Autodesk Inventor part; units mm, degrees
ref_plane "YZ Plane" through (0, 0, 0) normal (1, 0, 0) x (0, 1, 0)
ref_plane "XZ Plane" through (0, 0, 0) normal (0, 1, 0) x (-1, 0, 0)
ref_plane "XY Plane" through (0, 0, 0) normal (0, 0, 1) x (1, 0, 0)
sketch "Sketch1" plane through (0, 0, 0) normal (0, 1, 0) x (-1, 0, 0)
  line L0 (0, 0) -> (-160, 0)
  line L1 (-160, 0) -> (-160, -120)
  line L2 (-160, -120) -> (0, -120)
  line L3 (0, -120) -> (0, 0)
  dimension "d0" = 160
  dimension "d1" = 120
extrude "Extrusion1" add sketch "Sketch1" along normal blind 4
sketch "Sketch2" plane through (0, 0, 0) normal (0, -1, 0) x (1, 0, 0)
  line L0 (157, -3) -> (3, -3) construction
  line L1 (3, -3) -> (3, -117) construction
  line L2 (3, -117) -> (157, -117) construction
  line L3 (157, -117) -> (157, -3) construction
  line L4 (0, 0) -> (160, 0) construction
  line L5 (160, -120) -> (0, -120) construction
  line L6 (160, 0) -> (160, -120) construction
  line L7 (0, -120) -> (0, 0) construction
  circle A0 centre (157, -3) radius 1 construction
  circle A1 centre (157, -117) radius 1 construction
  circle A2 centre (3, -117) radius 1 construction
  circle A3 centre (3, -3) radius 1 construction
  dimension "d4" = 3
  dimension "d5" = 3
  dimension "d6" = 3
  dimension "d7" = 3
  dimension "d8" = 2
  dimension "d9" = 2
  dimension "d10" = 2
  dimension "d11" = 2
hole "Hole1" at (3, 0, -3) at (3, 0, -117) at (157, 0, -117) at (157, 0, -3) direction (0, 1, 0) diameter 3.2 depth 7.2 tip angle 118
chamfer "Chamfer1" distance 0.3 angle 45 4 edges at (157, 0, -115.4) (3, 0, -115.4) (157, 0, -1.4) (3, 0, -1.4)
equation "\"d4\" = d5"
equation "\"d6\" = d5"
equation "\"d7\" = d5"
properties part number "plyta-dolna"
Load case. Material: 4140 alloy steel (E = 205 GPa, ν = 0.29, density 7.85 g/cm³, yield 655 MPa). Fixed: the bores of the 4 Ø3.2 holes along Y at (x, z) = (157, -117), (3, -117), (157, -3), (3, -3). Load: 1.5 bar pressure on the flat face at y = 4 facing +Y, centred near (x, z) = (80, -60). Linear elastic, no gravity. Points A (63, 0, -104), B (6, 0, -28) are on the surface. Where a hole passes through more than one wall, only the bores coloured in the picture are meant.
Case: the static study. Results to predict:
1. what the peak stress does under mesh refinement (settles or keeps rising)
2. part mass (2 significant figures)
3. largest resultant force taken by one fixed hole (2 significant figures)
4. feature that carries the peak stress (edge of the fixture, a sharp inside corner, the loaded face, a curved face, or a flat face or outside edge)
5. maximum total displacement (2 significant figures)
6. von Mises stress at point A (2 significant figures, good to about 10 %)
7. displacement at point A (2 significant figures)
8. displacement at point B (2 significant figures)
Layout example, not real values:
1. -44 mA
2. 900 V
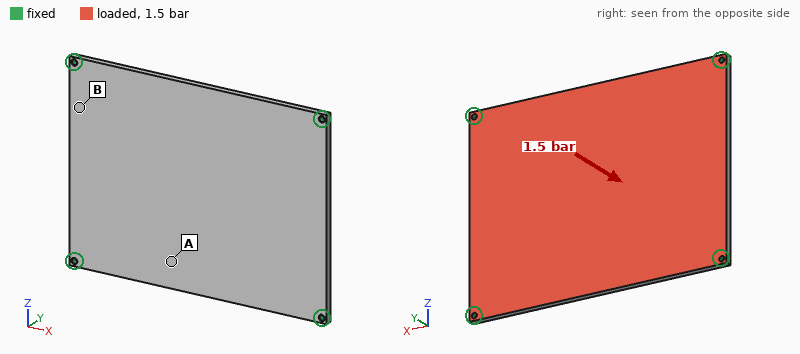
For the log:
1. keeps rising
2. 600 g
3. 720 N
4. edge of the fixture
5. 0.50 mm
6. 80 MPa
7. 0.42 mm
8. 0.095 mm
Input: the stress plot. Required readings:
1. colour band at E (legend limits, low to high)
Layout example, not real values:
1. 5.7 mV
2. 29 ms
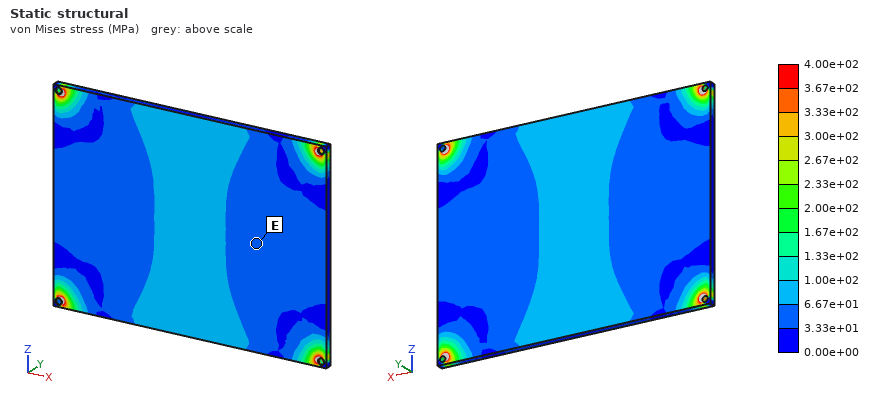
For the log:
1. 3.33e+01 to 6.67e+01 MPa
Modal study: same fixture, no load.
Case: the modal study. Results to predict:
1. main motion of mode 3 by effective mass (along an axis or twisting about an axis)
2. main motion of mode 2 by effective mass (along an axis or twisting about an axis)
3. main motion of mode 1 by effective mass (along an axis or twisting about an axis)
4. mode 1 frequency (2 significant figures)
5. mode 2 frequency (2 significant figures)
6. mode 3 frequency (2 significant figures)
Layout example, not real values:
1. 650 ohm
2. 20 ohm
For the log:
1. twisting about Z
2. twisting about X
3. along Y
4. 570 Hz
5. 1100 Hz
6. 1300 Hz
